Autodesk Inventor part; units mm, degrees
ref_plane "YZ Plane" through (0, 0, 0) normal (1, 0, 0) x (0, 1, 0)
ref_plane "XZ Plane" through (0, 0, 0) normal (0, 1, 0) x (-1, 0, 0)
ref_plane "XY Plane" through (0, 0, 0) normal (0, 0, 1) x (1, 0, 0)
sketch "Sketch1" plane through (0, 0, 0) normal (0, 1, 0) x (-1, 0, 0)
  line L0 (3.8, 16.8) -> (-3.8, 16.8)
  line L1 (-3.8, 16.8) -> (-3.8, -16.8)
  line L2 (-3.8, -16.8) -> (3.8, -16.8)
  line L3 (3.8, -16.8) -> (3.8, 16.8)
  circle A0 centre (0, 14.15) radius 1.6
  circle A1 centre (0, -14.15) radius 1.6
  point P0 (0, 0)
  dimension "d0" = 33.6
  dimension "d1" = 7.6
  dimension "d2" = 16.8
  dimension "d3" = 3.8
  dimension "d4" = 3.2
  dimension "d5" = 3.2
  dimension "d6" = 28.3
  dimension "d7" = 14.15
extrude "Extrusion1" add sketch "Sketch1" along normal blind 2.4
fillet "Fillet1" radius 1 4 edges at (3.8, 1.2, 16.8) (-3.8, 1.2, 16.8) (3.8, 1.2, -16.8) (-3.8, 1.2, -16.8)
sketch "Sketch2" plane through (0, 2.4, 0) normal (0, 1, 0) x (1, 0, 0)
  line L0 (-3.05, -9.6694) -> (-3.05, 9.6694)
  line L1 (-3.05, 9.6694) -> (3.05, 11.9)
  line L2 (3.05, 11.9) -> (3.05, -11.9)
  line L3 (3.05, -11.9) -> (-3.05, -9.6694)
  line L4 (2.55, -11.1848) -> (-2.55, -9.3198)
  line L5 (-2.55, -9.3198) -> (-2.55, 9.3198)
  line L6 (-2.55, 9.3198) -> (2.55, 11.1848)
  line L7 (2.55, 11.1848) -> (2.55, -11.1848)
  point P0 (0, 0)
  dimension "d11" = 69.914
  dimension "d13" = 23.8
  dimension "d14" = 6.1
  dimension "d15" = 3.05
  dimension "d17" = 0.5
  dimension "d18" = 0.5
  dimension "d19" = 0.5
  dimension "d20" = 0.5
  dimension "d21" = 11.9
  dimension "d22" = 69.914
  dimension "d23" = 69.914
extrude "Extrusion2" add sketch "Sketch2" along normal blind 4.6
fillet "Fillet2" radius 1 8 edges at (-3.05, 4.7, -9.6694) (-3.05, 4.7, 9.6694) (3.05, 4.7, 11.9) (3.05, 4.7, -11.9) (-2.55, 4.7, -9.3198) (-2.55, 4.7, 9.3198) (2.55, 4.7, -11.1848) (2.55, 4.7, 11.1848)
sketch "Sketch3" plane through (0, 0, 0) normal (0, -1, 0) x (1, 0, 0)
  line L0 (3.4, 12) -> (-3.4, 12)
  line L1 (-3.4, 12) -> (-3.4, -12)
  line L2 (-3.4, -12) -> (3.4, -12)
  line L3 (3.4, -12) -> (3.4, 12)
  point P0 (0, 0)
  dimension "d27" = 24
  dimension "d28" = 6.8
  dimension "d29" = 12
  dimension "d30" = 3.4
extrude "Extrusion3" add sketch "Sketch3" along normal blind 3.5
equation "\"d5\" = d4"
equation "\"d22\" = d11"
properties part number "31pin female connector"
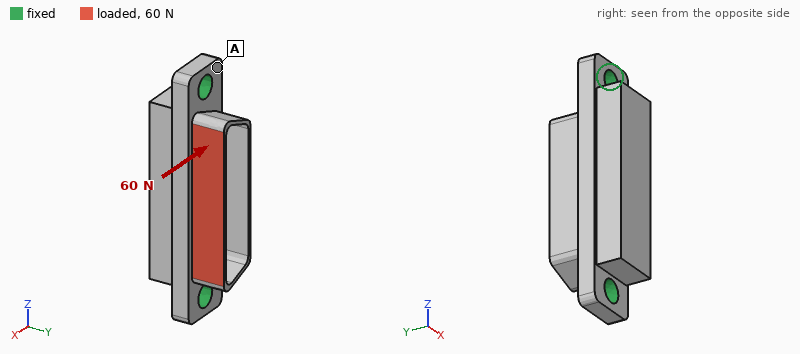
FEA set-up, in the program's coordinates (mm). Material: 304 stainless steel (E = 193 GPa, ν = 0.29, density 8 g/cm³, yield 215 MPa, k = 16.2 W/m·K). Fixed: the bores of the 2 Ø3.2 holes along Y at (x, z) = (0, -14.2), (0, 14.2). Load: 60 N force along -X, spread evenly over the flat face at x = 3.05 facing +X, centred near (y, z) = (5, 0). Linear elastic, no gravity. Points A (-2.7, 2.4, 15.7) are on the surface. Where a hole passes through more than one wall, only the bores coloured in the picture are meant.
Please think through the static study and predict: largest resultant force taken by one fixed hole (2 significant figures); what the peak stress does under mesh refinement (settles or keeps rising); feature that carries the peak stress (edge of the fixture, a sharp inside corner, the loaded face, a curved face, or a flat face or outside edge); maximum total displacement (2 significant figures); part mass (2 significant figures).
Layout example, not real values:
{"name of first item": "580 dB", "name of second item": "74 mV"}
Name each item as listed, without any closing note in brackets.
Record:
{"largest resultant force taken by one fixed hole": "30 N", "what the peak stress does under mesh refinement": "keeps rising", "feature that carries the peak stress": "a sharp inside corner", "maximum total displacement": "17 µm", "part mass": "10 g"}
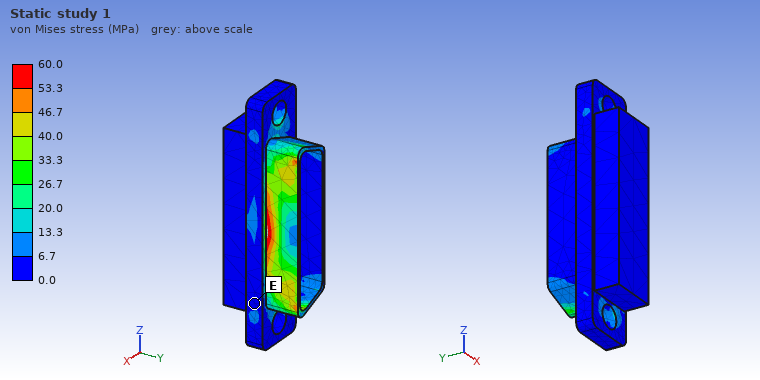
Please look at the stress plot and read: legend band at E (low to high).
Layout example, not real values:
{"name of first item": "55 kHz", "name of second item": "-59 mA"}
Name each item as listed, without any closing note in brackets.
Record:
{"legend band at E": "0.0 to 6.7 MPa"}
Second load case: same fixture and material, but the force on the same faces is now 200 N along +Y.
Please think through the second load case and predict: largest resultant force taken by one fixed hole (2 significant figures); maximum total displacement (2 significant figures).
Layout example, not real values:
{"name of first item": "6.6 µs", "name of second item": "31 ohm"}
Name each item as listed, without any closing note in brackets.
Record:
{"largest resultant force taken by one fixed hole": "110 N", "maximum total displacement": "9.9 µm"}
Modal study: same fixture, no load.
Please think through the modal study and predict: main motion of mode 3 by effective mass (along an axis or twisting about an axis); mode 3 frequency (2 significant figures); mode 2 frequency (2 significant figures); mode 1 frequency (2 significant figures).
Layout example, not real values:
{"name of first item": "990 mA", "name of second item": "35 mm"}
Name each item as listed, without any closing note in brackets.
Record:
{"main motion of mode 3 by effective mass": "along X", "mode 3 frequency": "23 kHz", "mode 2 frequency": "22 kHz", "mode 1 frequency": "20 kHz"}
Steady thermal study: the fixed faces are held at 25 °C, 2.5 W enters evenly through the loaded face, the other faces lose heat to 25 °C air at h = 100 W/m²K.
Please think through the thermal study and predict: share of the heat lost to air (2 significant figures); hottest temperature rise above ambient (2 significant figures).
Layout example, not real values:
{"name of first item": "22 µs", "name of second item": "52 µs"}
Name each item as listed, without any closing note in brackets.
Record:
{"share of the heat lost to air": "46 %", "hottest temperature rise above ambient": "43 K"}
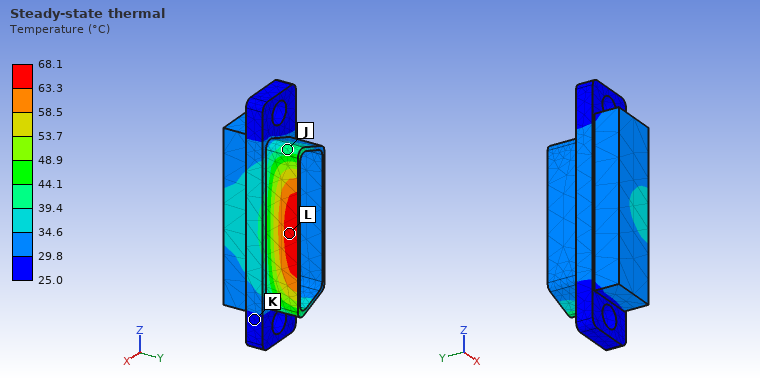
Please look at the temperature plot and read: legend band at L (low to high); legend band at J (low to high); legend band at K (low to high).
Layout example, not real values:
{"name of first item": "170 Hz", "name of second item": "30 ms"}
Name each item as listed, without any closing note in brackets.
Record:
{"legend band at L": "63.3 to 68.1 °C", "legend band at J": "39.4 to 44.1 °C", "legend band at K": "25.0 to 29.8 °C"}
